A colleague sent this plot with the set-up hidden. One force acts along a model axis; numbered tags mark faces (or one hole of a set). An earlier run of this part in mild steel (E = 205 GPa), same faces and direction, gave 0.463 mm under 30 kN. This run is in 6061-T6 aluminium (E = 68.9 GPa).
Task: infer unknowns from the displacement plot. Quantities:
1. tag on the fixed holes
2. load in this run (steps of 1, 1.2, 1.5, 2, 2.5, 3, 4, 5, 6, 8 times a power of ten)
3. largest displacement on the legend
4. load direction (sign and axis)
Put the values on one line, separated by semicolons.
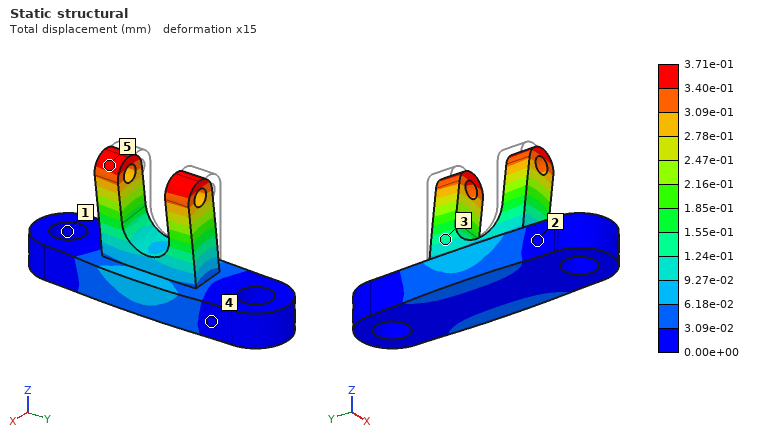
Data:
1; 8 kN; 3.71e-01 mm; +X
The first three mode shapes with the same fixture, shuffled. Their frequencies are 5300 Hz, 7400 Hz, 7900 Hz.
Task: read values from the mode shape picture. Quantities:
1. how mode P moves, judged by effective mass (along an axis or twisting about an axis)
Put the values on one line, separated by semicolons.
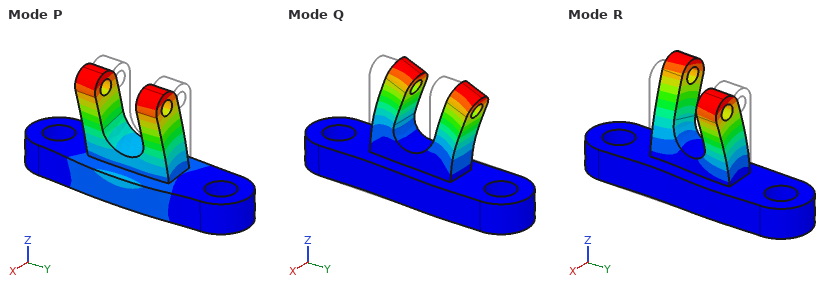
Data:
along X
